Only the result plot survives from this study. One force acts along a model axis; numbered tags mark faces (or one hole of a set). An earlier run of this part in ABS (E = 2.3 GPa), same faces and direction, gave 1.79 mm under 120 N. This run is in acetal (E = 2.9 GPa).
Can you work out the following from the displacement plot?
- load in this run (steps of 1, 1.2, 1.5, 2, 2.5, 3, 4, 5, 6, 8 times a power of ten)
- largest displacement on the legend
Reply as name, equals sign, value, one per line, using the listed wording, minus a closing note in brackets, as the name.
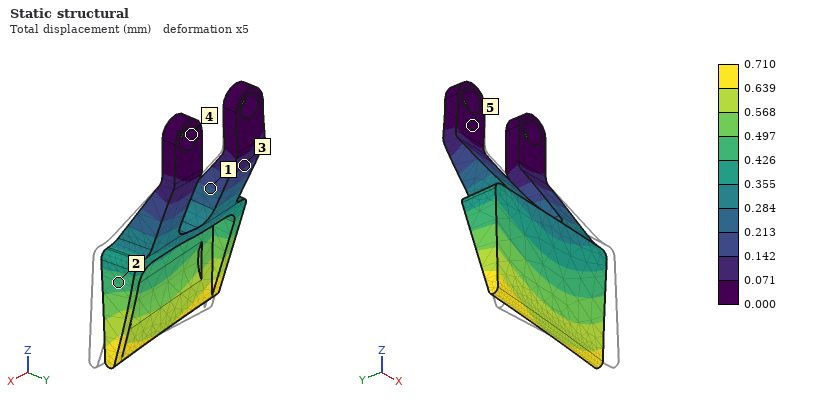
load in this run = 60 N
largest displacement on the legend = 0.710 mm
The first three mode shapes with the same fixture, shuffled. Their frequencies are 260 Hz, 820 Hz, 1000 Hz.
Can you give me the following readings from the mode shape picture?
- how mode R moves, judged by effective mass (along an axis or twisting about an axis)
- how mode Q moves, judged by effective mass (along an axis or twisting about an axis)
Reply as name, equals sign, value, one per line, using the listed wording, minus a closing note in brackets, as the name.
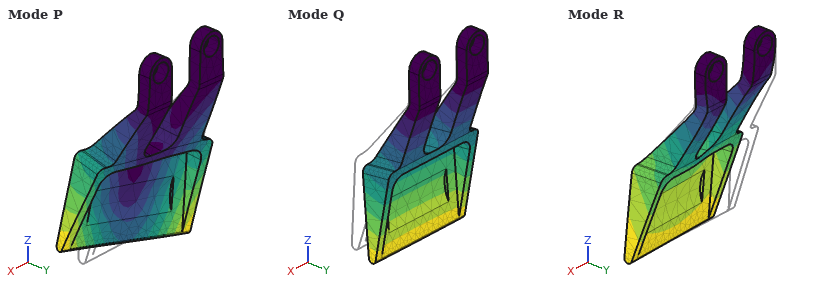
how mode R moves, judged by effective mass = along X
how mode Q moves, judged by effective mass = along Y
